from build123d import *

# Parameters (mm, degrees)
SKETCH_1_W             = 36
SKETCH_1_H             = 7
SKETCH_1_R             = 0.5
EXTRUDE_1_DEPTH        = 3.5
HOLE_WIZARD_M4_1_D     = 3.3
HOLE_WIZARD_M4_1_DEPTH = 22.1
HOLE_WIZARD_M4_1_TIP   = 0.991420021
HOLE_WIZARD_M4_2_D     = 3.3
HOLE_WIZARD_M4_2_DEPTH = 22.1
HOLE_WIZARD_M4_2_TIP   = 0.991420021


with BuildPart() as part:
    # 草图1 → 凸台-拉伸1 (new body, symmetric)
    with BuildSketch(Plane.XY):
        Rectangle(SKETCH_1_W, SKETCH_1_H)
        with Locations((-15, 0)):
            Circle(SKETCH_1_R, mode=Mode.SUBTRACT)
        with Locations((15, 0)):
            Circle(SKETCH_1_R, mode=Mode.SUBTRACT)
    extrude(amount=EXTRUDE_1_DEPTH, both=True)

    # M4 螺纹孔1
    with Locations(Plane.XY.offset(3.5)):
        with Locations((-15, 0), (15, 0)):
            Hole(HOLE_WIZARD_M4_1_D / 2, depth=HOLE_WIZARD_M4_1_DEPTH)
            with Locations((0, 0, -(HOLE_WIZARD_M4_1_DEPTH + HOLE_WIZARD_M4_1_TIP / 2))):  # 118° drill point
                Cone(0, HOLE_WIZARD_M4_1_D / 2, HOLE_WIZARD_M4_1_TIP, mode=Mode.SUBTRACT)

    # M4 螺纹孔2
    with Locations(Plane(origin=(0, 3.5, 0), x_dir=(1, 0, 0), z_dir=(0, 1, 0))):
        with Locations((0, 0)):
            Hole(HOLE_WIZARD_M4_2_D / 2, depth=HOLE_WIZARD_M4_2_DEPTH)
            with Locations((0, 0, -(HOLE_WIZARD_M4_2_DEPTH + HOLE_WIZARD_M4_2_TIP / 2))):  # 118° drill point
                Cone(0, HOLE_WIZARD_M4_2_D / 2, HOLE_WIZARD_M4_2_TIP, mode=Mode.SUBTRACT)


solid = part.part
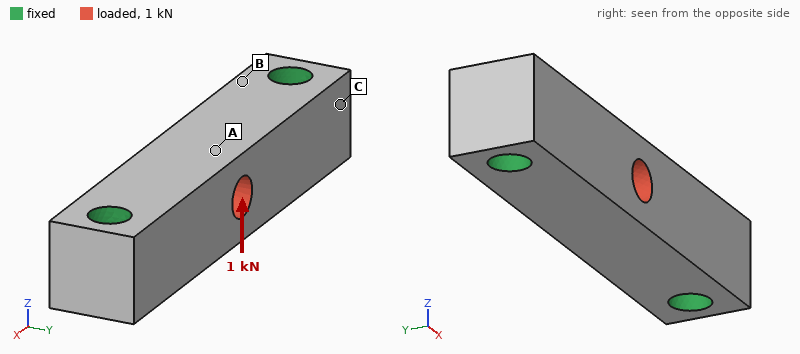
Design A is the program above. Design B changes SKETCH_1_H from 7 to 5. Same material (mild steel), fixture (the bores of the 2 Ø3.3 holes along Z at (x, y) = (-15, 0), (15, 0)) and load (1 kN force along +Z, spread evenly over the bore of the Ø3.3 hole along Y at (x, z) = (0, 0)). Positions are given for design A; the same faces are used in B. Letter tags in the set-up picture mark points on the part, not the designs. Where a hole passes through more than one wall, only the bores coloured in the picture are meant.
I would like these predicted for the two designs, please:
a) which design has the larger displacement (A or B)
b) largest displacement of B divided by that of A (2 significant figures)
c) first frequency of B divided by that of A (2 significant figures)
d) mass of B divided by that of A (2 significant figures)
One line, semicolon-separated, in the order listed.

B; 1.3; 0.88; 0.69
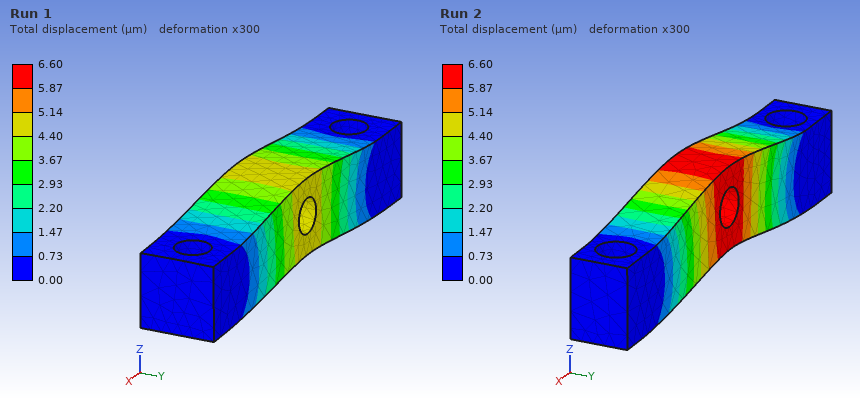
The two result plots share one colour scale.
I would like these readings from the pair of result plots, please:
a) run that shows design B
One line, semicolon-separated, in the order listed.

Run 2
